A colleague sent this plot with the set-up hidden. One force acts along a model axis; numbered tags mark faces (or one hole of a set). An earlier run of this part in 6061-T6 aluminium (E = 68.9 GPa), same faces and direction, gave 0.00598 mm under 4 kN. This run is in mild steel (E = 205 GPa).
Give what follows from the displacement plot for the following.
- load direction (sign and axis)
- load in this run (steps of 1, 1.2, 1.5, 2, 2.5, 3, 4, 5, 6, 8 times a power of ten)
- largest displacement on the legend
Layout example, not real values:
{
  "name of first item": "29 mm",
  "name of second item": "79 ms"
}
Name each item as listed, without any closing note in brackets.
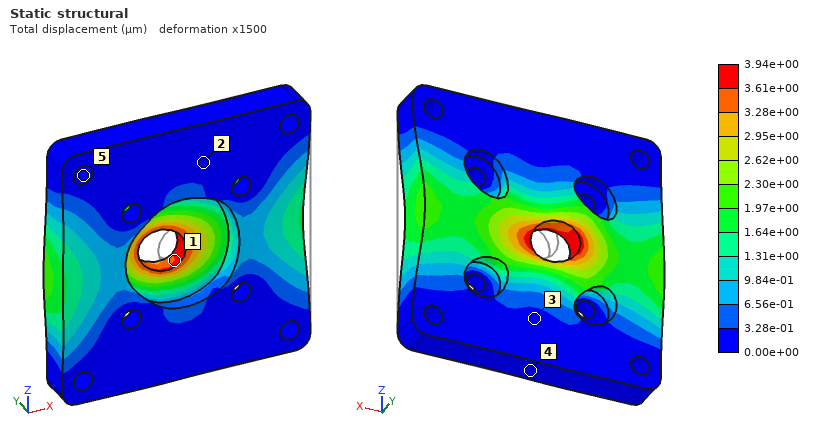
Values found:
{
  "load direction": "-X",
  "load in this run": "8 kN",
  "largest displacement on the legend": "3.94e+00 µm"
}
